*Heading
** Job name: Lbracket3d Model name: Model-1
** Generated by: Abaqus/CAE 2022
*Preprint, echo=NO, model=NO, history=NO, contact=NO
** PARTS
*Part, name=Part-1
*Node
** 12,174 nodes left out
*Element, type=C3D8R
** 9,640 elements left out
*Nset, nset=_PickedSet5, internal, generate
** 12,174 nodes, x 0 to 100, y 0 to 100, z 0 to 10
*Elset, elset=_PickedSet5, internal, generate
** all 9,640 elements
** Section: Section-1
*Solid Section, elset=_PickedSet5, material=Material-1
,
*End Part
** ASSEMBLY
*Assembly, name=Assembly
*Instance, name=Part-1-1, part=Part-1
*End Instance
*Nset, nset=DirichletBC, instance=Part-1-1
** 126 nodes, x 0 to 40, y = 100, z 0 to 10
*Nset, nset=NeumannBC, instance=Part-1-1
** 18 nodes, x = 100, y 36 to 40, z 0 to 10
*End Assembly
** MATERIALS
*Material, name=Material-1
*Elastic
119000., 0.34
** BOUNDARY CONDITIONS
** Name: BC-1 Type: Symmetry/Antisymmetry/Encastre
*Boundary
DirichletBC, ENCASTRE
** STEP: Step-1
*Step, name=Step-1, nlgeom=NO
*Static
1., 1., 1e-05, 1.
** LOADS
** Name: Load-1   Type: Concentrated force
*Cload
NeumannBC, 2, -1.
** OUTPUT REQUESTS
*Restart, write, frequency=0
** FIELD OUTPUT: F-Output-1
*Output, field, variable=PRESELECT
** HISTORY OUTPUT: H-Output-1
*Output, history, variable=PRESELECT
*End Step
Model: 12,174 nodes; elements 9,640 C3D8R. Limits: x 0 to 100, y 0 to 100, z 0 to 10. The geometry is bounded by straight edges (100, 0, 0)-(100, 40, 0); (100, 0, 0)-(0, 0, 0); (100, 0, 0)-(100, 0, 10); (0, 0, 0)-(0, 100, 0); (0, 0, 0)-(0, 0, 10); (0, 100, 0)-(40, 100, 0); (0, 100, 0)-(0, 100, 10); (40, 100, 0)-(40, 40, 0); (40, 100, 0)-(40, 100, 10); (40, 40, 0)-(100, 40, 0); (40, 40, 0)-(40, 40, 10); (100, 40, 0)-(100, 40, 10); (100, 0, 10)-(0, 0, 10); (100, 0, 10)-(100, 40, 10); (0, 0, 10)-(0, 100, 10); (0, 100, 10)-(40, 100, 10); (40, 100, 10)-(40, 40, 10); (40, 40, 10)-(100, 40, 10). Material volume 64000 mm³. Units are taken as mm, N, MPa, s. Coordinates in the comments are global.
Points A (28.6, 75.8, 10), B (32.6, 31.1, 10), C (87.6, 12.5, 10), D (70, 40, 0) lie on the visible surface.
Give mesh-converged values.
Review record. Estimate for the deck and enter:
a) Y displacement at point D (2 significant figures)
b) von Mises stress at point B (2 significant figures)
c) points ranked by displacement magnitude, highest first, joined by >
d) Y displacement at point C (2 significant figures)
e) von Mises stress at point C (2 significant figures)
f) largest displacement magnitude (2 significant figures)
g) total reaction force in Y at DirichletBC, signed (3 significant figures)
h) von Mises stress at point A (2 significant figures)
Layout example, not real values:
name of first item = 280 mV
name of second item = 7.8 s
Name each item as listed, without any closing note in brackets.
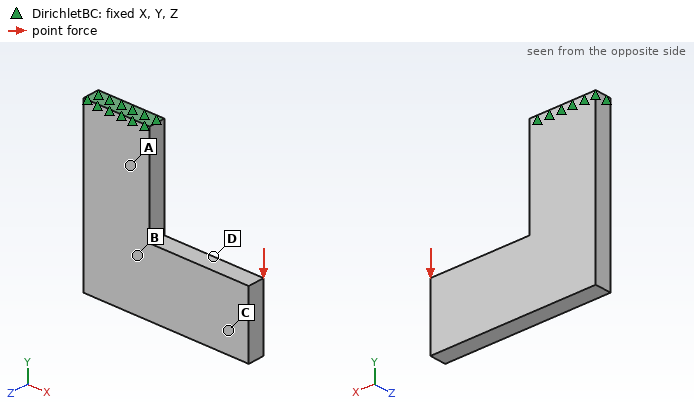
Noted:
Y displacement at point D = -0.0010 mm
von Mises stress at point B = 0.24 MPa
points ranked by displacement magnitude, highest first, joined by > = C > D > B > A
Y displacement at point C = -0.0015 mm
von Mises stress at point C = 0.12 MPa
largest displacement magnitude = 0.0021 mm
total reaction force in Y at DirichletBC, signed = 18.0 N
von Mises stress at point A = 0.28 MPa
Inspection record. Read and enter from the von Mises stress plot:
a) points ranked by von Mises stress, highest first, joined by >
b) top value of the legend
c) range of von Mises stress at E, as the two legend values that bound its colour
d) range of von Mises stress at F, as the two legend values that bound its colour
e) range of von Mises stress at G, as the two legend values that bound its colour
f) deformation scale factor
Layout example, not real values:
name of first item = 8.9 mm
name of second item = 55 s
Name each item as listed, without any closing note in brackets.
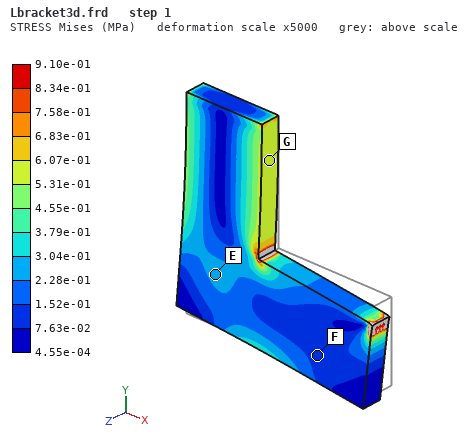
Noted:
points ranked by von Mises stress, highest first, joined by > = G > E > F
top value of the legend = 9.10e-01 MPa
range of von Mises stress at E, as the two legend values that bound its colour = 2.28e-01 to 3.04e-01 MPa
range of von Mises stress at F, as the two legend values that bound its colour = 7.63e-02 to 1.52e-01 MPa
range of von Mises stress at G, as the two legend values that bound its colour = 5.31e-01 to 6.07e-01 MPa
deformation scale factor = 5000
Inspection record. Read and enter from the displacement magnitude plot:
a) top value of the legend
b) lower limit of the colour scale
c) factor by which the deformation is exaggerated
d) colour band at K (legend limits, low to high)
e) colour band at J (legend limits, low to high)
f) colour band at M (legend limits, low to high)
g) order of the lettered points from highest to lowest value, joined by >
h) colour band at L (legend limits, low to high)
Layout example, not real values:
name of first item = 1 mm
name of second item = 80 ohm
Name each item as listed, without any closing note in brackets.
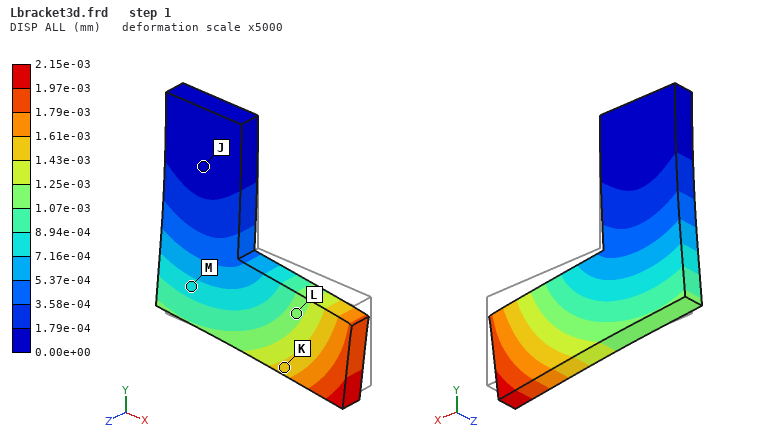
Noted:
top value of the legend = 2.15e-03 mm
lower limit of the colour scale = 0.00e+00 mm
factor by which the deformation is exaggerated = 5000
colour band at K = 1.43e-03 to 1.61e-03 mm
colour band at J = 0.00e+00 to 1.79e-04 mm
colour band at M = 7.16e-04 to 8.94e-04 mm
order of the lettered points from highest to lowest value, joined by > = K > L > M > J
colour band at L = 1.07e-03 to 1.25e-03 mm
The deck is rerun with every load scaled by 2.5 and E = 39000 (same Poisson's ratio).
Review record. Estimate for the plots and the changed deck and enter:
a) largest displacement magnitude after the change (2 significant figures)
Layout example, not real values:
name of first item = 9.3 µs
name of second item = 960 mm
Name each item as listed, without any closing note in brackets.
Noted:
largest displacement magnitude after the change = 0.016 mm
